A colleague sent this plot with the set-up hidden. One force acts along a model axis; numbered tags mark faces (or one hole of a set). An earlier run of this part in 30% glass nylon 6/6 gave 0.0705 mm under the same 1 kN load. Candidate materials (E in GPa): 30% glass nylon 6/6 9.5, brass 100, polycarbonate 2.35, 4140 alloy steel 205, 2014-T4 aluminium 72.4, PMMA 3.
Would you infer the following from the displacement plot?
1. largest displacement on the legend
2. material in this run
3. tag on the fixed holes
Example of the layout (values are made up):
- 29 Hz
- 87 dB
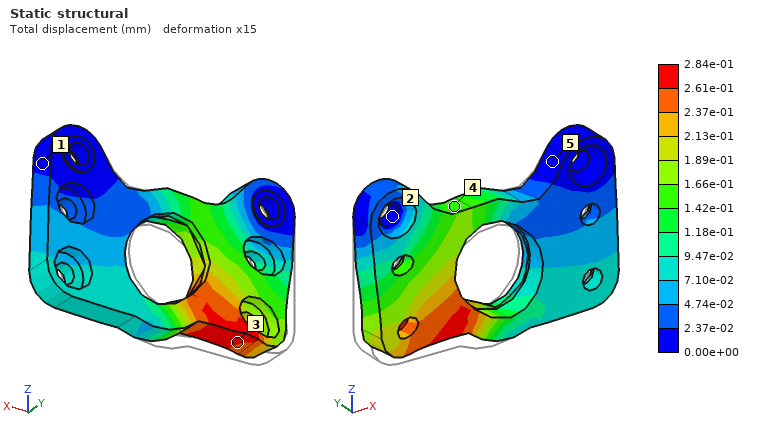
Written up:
- 2.84e-01 mm
- polycarbonate
- 2
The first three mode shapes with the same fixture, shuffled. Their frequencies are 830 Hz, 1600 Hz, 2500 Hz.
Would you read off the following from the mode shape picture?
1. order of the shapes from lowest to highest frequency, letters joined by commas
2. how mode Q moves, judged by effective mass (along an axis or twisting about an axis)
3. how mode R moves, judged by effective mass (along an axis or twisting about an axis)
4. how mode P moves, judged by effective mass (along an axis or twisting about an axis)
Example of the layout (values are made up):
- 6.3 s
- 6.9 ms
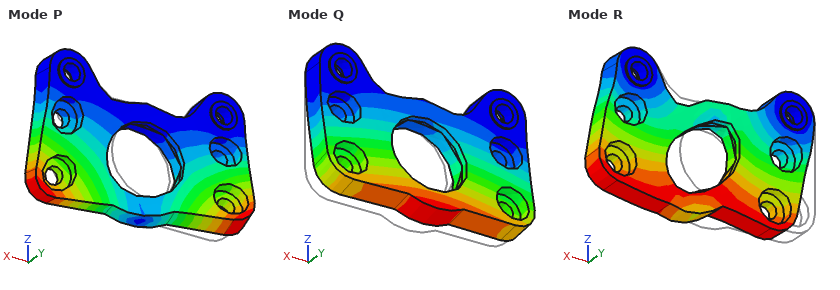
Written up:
- Q, P, R
- along Y
- along X
- twisting about Z
